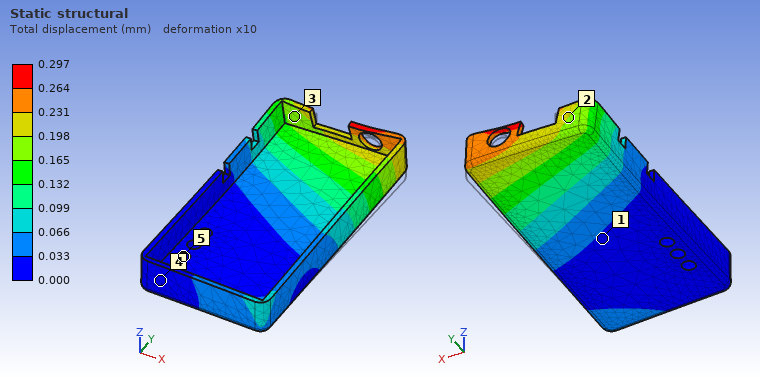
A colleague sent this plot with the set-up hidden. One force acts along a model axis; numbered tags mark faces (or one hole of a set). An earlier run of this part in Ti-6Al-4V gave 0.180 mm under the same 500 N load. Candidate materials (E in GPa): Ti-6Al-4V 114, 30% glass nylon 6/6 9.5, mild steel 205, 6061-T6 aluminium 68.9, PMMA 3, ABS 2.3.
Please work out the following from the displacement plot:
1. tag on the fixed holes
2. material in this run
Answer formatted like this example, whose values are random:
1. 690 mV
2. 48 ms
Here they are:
1. 5
2. 6061-T6 aluminium
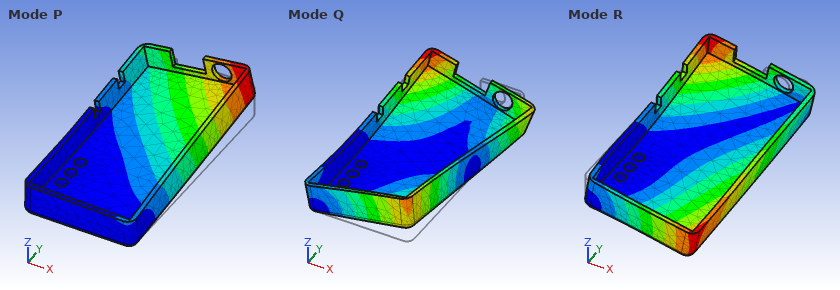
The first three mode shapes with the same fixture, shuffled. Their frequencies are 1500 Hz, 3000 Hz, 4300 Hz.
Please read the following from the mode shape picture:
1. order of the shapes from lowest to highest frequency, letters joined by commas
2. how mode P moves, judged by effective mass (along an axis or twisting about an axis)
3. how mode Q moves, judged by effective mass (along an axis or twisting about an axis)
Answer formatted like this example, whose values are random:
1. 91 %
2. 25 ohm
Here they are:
1. P, R, Q
2. along Z
3. along Z
